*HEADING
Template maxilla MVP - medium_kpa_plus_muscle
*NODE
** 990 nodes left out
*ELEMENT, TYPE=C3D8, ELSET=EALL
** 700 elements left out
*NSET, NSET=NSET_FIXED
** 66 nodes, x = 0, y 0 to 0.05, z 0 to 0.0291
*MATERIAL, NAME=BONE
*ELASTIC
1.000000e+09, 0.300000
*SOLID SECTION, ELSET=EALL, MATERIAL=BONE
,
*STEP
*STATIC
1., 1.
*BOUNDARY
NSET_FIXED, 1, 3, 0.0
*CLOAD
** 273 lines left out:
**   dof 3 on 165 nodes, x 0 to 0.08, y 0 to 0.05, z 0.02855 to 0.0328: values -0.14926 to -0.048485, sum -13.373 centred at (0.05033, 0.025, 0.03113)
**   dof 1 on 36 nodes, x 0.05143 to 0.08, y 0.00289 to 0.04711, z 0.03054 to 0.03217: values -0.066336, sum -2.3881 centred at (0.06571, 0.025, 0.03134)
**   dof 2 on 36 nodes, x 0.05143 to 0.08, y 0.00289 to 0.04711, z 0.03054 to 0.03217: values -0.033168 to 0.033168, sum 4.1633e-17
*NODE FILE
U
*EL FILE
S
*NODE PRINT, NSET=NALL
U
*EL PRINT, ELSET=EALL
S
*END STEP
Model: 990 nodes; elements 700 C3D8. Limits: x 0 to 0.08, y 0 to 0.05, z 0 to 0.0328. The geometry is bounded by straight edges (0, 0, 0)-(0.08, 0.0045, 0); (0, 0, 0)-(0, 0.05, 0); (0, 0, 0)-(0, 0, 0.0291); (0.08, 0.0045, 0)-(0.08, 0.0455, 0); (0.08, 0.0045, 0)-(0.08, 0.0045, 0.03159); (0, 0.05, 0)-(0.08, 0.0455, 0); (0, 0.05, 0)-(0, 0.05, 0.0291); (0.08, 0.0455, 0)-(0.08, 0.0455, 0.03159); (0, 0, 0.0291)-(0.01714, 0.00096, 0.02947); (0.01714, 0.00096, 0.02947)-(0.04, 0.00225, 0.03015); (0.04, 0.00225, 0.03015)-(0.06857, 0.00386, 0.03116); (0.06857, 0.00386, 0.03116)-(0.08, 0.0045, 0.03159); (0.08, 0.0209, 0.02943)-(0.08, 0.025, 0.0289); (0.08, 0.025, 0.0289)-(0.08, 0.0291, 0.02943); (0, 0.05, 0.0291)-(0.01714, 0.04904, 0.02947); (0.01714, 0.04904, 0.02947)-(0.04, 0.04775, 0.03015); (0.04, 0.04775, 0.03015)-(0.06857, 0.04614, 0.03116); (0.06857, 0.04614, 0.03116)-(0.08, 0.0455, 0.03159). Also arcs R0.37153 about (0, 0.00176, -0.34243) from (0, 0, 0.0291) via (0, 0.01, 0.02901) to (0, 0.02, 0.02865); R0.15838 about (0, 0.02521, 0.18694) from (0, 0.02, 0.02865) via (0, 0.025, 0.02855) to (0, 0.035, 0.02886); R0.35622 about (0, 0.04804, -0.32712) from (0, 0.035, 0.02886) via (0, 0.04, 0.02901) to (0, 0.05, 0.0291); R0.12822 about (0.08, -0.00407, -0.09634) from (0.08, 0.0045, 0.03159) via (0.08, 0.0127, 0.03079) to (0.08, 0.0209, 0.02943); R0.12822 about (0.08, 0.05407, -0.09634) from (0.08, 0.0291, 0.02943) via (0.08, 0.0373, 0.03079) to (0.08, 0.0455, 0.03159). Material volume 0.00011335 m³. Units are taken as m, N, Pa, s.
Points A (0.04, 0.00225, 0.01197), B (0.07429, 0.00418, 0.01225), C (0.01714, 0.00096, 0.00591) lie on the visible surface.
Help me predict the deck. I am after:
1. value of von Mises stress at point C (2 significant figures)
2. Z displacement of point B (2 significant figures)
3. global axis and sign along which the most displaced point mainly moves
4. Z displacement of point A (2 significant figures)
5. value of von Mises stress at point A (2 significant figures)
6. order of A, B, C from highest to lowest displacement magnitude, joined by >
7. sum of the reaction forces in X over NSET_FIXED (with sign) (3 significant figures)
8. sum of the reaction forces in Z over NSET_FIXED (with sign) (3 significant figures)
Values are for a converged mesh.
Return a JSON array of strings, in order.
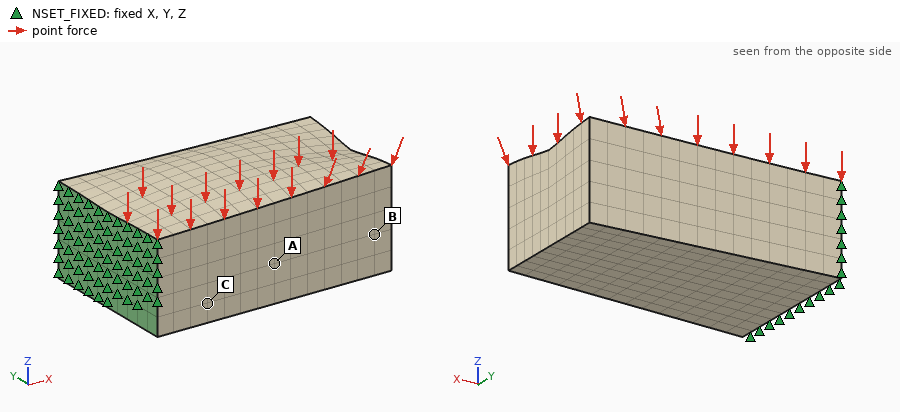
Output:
["37000 Pa", "-1.0e-05 m", "-Z", "-4.2e-06 m", "22000 Pa", "B > A > C", "2.39 N", "13.4 N"]
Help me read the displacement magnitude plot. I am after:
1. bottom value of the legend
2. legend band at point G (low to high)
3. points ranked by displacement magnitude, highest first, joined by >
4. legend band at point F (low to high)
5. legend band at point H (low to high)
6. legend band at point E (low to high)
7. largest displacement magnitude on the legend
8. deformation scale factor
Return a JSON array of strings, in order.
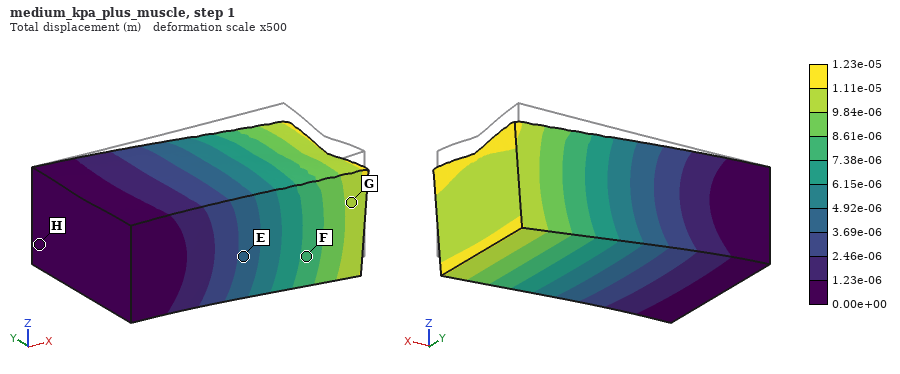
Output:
["0.00e+00 m", "9.84e-06 to 1.11e-05 m", "G > F > E > H", "7.38e-06 to 8.61e-06 m", "0.00e+00 to 1.23e-06 m", "3.69e-06 to 4.92e-06 m", "1.23e-05 m", "500"]
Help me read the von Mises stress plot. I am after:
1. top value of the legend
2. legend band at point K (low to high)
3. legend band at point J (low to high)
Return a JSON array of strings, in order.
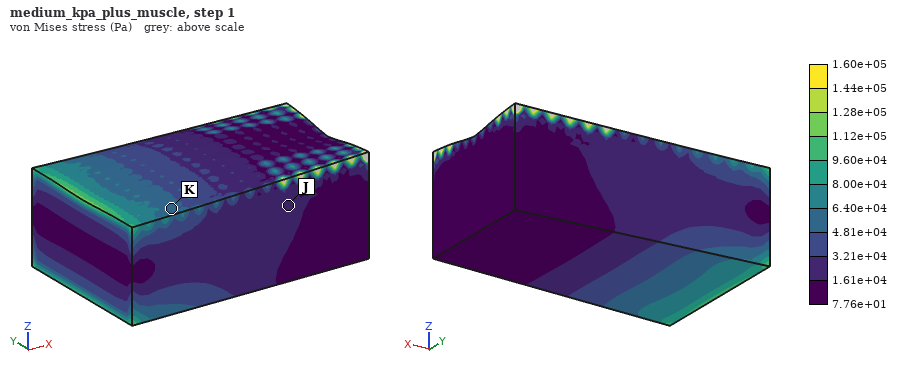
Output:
["1.60e+05 Pa", "4.81e+04 to 6.40e+04 Pa", "1.61e+04 to 3.21e+04 Pa"]
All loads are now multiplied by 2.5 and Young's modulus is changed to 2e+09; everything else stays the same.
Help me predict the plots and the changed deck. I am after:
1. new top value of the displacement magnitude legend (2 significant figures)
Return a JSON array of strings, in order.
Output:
["1.5e-05 m"]
